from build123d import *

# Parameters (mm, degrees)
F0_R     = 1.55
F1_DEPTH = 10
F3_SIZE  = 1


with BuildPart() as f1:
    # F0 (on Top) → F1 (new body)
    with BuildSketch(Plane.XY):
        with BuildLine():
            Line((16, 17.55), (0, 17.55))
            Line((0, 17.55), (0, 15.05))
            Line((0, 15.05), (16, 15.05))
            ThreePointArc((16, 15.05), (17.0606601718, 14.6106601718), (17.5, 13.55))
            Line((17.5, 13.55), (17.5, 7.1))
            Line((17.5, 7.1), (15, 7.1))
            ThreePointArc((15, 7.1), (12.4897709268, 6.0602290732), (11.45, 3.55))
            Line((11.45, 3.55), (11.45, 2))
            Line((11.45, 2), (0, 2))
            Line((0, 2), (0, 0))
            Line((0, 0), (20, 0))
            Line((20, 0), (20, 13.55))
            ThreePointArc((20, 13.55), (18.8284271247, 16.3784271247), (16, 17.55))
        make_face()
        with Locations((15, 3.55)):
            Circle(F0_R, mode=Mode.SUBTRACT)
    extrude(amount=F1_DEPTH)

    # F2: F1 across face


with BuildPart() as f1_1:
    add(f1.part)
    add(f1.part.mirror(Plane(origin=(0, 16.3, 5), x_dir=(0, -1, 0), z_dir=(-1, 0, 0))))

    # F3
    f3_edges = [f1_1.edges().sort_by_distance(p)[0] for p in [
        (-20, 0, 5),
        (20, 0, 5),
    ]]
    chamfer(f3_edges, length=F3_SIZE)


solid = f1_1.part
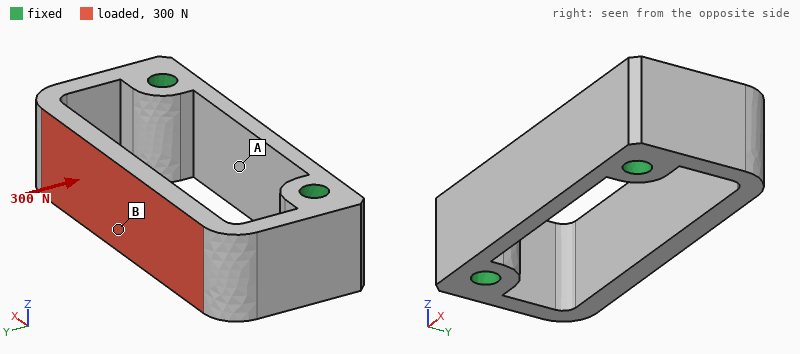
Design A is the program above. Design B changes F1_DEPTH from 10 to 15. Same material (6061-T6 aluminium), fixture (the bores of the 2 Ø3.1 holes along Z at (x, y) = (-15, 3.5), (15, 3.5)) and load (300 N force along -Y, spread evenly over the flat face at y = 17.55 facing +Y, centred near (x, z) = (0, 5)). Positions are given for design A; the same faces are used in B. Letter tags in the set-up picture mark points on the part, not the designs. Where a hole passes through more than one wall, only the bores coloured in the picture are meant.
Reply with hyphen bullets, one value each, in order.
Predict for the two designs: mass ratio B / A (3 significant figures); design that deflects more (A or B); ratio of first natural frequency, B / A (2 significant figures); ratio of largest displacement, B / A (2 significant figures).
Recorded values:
- 1.50
- A
- 1.0
- 0.67
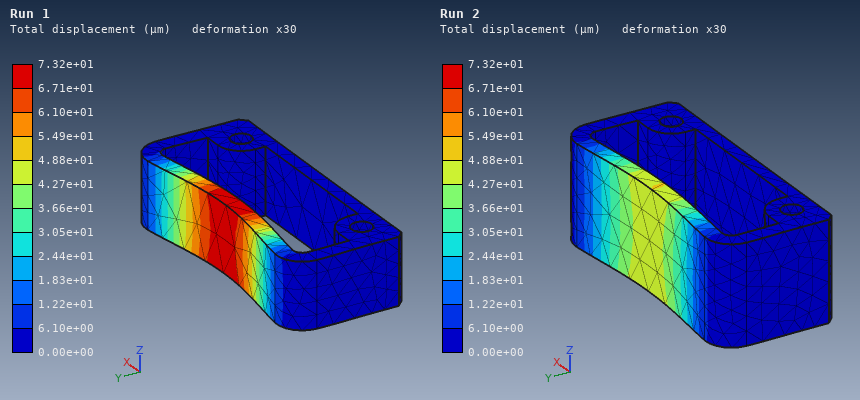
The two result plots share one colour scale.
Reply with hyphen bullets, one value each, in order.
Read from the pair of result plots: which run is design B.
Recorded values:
- Run 2
